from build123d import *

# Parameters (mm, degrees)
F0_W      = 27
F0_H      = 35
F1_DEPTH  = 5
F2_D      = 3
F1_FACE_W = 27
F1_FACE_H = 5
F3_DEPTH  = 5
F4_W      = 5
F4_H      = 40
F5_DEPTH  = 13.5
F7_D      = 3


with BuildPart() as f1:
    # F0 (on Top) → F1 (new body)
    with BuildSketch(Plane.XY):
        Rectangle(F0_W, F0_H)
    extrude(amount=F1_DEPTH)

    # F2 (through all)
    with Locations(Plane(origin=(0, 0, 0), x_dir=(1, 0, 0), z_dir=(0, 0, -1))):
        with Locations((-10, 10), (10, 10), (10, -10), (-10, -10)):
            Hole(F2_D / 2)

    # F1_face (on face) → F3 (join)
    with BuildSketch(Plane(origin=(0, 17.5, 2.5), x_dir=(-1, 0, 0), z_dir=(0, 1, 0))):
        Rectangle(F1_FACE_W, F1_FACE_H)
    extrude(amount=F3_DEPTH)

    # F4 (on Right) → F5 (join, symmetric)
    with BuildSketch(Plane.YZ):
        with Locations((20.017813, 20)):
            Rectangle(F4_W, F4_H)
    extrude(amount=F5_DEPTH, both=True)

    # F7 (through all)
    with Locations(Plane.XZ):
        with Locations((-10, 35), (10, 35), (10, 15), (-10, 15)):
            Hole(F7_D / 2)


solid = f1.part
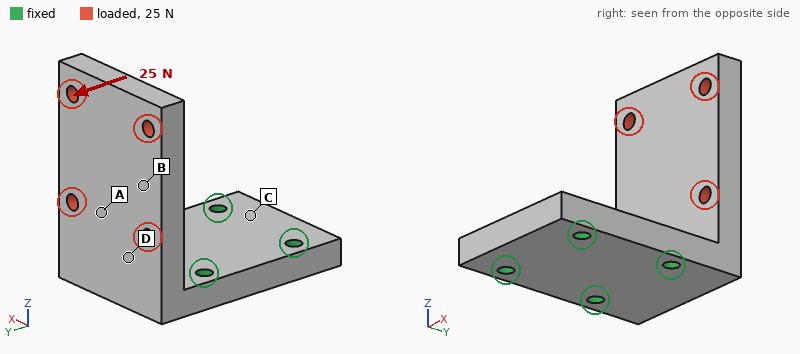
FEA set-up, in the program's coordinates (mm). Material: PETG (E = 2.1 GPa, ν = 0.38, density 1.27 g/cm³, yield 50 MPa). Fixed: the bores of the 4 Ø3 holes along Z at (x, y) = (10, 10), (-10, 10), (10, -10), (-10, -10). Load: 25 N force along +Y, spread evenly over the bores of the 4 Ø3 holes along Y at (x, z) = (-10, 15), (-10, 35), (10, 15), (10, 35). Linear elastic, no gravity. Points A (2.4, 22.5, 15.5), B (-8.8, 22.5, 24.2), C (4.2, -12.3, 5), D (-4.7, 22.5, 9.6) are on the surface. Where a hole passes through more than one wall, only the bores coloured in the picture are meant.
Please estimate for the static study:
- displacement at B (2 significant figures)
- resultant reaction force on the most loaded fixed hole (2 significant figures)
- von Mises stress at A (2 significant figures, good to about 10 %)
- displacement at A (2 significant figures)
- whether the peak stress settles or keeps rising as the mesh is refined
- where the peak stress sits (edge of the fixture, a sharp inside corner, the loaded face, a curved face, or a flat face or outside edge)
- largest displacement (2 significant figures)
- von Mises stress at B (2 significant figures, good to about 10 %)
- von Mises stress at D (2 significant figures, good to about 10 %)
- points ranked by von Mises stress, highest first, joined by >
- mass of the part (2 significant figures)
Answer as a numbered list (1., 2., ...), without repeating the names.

1. 0.33 mm
2. 12 N
3. 2.2 MPa
4. 0.19 mm
5. keeps rising
6. edge of the fixture
7. 0.64 mm
8. 1.2 MPa
9. 3.2 MPa
10. D > A > B > C
11. 13 g
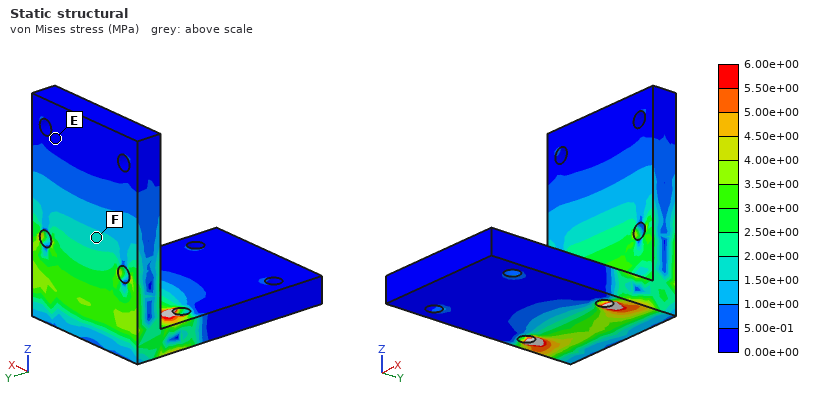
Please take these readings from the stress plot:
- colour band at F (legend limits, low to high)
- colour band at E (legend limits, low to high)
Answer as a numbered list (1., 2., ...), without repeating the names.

1. 1.50e+00 to 2.00e+00 MPa
2. 0.00e+00 to 5.00e-01 MPa
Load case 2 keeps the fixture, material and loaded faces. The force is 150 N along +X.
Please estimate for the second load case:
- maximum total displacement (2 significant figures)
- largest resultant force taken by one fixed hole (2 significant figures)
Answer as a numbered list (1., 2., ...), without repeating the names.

1. 0.65 mm
2. 190 N
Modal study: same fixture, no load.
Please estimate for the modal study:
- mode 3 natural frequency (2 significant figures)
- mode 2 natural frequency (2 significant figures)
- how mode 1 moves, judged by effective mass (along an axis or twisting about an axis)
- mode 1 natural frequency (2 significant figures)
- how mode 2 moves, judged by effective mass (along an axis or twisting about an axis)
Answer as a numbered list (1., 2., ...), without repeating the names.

1. 2100 Hz
2. 1300 Hz
3. along Y
4. 540 Hz
5. along X
